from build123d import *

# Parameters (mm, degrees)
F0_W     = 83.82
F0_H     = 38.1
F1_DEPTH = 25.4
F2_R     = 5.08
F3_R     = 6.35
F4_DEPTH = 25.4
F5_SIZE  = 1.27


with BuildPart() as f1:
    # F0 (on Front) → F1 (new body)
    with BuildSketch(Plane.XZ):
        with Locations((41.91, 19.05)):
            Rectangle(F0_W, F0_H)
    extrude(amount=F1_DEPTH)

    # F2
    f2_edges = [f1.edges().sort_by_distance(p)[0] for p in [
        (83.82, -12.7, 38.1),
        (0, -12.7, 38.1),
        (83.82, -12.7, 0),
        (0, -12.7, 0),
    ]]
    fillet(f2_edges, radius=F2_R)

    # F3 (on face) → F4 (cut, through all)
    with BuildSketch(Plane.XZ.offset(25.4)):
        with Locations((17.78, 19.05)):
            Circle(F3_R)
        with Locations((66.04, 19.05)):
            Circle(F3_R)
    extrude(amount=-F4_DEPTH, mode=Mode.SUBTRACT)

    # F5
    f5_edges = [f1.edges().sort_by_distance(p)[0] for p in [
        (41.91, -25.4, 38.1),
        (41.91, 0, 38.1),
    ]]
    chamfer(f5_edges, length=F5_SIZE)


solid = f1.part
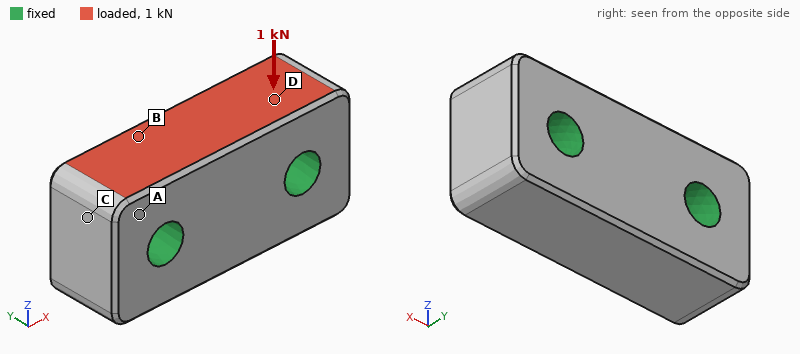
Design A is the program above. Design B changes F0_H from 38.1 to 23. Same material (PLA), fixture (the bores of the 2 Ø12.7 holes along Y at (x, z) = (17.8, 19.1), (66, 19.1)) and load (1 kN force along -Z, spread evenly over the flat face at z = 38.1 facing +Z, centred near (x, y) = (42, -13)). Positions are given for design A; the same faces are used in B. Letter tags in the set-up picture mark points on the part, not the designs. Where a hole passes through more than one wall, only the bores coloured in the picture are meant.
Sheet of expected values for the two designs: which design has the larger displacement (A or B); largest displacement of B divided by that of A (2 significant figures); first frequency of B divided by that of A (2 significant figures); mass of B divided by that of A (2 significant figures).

B
1.3
1.1
0.56
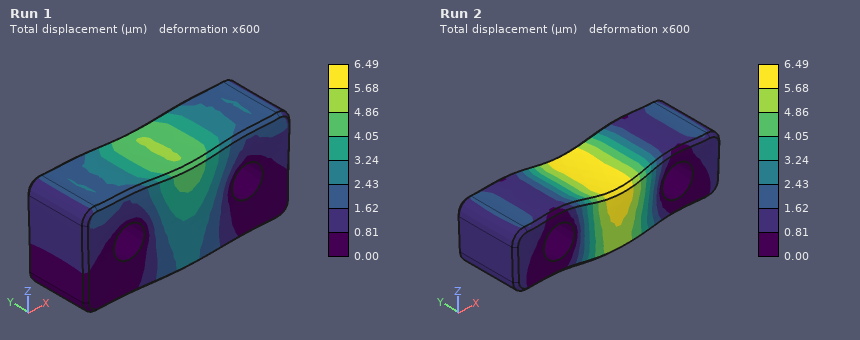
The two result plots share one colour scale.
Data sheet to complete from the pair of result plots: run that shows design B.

Run 2
